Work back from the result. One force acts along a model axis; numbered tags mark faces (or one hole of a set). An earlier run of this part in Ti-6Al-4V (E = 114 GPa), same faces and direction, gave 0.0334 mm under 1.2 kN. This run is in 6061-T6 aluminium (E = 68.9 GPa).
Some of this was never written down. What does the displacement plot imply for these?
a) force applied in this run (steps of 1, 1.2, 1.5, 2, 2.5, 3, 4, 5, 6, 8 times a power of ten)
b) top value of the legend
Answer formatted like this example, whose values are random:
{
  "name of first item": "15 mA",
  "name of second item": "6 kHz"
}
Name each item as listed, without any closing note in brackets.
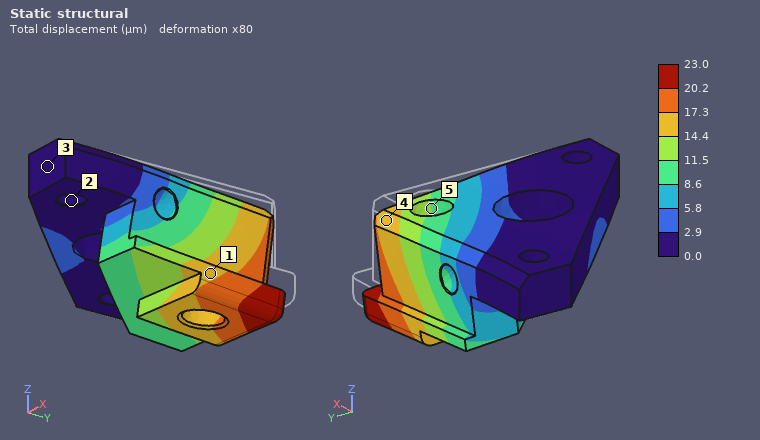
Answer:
{
  "force applied in this run": "500 N",
  "top value of the legend": "23.0 µm"
}
